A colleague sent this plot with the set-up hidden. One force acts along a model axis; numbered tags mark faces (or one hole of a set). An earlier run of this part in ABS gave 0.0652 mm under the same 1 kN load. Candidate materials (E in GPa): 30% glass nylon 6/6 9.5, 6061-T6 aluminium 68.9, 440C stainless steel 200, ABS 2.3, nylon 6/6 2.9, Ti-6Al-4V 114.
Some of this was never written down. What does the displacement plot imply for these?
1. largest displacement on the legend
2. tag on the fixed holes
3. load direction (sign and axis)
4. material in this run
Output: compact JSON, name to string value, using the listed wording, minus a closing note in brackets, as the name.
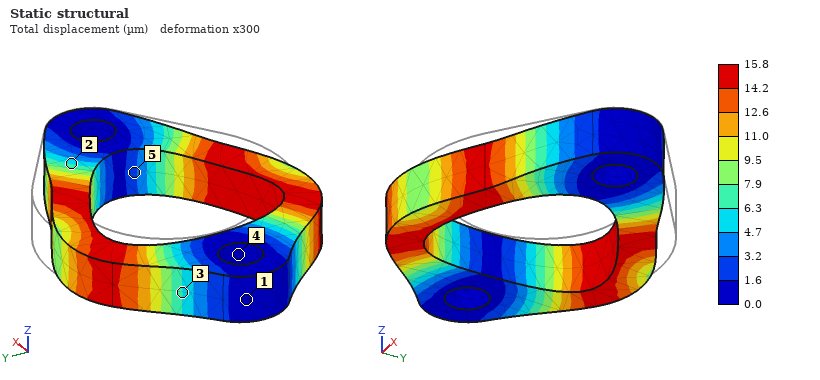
{"largest displacement on the legend": "15.8 µm", "tag on the fixed holes": "4", "load direction": "-X", "material in this run": "30% glass nylon 6/6"}
